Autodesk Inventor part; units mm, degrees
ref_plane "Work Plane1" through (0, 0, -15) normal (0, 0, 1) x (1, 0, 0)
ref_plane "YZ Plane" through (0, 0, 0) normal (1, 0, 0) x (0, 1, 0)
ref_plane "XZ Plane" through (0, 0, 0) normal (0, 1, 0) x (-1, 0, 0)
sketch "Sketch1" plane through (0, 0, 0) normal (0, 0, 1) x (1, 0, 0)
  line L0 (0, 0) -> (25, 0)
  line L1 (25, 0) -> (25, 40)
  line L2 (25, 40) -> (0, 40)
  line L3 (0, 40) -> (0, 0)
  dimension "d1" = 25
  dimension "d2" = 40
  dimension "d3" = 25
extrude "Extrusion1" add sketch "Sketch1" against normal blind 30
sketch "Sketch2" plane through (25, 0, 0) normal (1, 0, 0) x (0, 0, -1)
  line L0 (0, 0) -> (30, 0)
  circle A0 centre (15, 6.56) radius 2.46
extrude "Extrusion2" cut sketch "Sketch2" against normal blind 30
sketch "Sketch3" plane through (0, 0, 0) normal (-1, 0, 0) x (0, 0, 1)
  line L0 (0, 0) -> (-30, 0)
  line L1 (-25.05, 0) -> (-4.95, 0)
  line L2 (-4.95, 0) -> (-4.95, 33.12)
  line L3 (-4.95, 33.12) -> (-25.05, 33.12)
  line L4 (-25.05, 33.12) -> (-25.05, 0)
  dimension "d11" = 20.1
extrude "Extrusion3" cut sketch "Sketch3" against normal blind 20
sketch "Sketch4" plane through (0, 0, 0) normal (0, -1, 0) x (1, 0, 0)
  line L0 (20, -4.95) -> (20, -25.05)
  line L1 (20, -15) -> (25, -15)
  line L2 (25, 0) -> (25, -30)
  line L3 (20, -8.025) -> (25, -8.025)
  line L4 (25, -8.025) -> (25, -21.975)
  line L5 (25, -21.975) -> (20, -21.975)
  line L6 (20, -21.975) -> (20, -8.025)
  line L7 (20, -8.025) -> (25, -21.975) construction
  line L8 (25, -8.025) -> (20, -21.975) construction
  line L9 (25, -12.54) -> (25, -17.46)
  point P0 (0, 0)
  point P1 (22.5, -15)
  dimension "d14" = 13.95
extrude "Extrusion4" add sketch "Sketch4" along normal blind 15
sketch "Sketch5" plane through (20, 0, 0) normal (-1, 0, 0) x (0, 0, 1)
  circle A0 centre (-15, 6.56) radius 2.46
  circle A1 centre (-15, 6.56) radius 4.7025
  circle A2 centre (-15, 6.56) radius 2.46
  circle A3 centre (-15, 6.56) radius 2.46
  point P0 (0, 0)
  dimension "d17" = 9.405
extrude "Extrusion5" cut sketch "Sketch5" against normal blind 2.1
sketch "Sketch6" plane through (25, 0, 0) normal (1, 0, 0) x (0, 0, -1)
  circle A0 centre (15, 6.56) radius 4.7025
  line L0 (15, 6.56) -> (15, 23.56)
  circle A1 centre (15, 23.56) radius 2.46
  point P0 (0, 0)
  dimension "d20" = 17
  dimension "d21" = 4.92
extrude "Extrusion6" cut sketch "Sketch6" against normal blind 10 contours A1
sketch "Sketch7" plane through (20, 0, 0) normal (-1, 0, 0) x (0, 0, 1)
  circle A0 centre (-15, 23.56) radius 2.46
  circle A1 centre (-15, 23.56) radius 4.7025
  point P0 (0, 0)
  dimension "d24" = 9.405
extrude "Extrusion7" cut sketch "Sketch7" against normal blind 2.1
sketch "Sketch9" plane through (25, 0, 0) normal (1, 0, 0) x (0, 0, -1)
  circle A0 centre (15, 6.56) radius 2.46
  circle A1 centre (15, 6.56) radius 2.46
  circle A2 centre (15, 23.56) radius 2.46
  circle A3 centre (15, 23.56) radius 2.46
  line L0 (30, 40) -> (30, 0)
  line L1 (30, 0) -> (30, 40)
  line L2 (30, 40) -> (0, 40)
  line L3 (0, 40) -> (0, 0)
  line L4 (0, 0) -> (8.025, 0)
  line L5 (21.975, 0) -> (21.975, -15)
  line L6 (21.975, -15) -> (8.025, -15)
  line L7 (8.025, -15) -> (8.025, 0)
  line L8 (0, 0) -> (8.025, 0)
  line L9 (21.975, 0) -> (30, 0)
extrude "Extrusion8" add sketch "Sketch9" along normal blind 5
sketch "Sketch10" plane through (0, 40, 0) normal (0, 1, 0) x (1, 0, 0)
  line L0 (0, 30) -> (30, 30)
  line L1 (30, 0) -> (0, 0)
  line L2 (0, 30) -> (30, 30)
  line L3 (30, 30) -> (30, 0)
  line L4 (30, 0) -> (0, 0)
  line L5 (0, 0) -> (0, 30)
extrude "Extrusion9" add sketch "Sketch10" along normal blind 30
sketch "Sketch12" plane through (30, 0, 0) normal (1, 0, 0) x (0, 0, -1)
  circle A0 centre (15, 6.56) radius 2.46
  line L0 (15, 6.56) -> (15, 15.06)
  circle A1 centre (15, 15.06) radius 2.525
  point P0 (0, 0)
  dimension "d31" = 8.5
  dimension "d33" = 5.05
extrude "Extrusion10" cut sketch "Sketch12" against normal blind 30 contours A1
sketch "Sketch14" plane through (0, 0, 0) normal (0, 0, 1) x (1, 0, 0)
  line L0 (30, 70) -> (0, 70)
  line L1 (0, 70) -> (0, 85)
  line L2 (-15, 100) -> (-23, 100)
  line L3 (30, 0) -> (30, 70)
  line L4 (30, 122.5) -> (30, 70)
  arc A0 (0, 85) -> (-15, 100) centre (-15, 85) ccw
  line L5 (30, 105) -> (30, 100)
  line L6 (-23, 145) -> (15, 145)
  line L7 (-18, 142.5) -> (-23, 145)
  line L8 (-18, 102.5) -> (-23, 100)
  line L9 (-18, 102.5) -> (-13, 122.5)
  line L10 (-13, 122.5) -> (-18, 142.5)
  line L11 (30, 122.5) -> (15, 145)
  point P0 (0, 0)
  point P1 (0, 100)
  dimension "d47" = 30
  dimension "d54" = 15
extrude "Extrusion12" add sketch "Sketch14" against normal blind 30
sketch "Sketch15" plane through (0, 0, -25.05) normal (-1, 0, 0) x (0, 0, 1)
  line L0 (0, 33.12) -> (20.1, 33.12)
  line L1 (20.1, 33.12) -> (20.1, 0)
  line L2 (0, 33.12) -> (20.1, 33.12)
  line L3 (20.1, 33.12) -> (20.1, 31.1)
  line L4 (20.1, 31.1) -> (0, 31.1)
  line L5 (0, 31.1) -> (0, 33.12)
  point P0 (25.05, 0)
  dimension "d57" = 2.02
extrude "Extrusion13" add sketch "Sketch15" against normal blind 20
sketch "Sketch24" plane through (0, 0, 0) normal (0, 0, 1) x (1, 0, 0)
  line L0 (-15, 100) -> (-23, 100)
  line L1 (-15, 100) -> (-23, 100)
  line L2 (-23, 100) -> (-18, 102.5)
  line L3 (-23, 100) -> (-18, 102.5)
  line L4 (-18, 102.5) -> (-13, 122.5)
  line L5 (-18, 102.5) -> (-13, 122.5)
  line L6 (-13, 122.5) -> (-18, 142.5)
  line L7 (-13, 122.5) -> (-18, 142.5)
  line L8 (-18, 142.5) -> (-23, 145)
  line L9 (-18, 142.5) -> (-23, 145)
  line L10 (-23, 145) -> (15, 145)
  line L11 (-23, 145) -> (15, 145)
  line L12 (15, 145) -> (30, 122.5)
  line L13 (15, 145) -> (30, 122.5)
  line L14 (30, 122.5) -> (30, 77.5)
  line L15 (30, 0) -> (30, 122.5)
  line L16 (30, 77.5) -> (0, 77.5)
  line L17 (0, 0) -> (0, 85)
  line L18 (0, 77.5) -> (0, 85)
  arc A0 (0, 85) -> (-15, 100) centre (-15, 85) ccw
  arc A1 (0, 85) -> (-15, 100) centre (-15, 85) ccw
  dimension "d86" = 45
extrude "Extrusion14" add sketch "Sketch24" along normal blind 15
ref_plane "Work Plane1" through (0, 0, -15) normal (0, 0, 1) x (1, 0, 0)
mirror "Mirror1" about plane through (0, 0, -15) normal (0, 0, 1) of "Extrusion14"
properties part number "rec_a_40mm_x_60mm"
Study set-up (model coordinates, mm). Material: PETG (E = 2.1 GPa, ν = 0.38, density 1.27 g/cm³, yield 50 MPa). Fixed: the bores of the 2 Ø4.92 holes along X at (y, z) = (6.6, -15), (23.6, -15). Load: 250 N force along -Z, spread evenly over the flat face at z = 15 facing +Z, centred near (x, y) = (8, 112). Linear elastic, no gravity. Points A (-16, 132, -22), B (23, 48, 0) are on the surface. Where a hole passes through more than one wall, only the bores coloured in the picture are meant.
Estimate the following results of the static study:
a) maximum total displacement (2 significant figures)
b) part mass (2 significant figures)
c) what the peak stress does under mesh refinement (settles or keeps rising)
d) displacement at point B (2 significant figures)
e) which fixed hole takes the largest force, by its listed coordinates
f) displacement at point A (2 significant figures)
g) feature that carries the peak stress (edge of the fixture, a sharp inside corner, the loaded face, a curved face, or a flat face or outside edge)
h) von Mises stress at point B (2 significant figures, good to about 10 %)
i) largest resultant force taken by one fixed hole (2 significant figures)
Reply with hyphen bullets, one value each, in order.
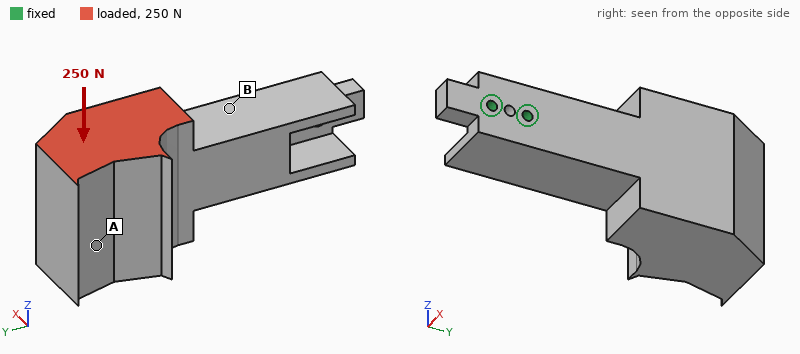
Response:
- 2.1 mm
- 270 g
- keeps rising
- 0.36 mm
- (23.6, -15)
- 1.8 mm
- edge of the fixture
- 4.1 MPa
- 1.2 kN
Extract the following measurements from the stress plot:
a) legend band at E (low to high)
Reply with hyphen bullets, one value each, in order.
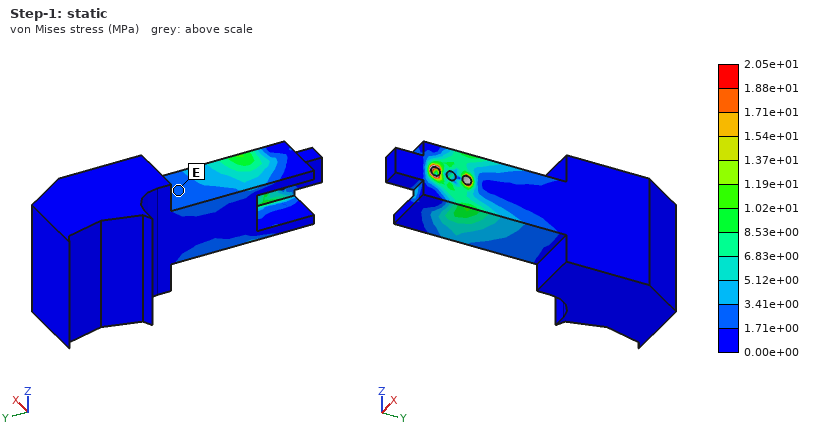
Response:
- 1.71e+00 to 3.41e+00 MPa
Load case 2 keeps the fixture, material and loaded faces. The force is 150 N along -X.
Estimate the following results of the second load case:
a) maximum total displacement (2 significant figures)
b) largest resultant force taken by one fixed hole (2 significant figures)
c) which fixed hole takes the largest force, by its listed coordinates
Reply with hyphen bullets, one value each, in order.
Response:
- 1.9 mm
- 680 N
- (23.6, -15)
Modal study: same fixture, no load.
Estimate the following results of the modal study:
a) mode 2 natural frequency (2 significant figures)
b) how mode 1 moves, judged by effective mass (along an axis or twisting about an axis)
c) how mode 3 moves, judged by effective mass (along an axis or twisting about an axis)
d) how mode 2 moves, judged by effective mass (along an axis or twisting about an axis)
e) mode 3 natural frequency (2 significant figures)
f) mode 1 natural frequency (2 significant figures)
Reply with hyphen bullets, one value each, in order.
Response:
- 140 Hz
- along X
- twisting about Y
- along Z
- 350 Hz
- 120 Hz
